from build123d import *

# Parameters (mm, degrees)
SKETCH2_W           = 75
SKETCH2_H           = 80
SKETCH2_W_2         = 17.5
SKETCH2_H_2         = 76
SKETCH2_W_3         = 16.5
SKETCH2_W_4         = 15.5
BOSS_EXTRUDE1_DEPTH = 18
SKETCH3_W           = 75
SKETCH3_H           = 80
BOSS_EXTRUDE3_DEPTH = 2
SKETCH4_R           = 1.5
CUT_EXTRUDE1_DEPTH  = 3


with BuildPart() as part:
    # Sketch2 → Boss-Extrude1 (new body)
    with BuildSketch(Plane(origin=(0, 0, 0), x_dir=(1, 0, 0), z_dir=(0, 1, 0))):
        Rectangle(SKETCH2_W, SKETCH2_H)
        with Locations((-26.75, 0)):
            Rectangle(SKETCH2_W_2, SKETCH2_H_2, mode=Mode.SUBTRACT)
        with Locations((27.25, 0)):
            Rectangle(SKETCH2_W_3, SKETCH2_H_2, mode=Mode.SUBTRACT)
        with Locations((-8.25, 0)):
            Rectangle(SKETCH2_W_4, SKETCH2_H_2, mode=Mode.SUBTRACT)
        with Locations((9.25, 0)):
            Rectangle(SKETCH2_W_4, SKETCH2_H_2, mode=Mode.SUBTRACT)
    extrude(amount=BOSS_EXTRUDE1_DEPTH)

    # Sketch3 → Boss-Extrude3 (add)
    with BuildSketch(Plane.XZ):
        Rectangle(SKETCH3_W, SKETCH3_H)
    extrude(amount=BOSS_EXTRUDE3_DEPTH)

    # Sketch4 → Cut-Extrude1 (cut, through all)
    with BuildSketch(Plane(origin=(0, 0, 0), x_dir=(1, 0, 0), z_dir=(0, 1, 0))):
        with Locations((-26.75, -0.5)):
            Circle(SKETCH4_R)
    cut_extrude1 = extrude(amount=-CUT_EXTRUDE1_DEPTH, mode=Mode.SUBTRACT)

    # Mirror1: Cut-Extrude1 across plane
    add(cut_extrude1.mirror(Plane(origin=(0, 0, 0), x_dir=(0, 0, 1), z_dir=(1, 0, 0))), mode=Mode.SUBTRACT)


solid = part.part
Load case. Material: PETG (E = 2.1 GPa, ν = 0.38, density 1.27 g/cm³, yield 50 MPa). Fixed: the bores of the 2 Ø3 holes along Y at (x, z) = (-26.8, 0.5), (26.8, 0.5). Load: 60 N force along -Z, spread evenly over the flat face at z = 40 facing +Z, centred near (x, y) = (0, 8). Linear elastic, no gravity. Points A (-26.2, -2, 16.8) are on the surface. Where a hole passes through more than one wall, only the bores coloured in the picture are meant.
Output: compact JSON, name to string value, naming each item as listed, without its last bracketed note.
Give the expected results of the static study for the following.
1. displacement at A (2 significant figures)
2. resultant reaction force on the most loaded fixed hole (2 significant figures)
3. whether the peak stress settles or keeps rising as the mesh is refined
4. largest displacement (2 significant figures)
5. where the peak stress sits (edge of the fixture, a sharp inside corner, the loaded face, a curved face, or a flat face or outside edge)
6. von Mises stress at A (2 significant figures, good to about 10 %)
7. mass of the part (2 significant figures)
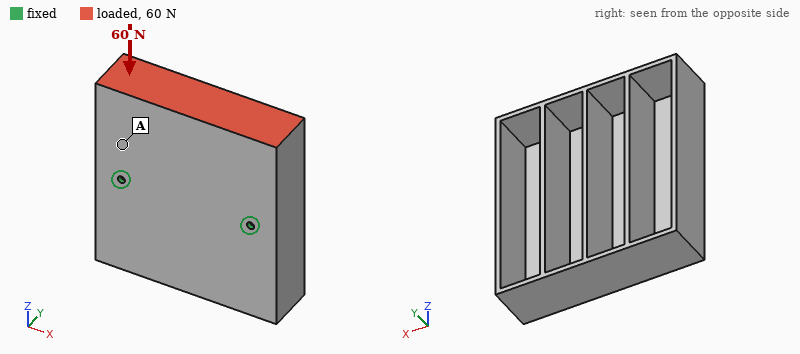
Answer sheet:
{"displacement at A": "0.35 mm", "resultant reaction force on the most loaded fixed hole": "30 N", "whether the peak stress settles or keeps rising as the mesh is refined": "keeps rising", "largest displacement": "1.0 mm", "where the peak stress sits": "edge of the fixture", "von Mises stress at A": "1.2 MPa", "mass of the part": "39 g"}
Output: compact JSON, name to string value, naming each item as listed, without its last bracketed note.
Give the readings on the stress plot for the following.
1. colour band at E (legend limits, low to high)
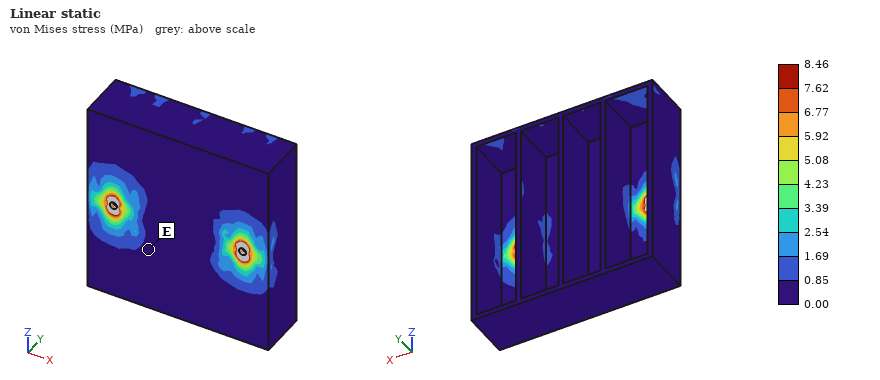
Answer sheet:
{"colour band at E": "0.00 to 0.85 MPa"}
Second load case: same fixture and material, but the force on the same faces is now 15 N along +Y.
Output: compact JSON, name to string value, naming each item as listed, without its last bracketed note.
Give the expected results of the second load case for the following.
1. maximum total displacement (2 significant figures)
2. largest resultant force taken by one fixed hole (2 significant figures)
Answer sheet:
{"maximum total displacement": "1.1 mm", "largest resultant force taken by one fixed hole": "7.6 N"}
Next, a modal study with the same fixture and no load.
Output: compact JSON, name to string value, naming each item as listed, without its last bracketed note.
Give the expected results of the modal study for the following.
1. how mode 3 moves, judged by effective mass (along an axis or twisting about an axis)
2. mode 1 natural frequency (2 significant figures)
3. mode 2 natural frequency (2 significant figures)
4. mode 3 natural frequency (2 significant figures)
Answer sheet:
{"how mode 3 moves, judged by effective mass": "along Y", "mode 1 natural frequency": "140 Hz", "mode 2 natural frequency": "310 Hz", "mode 3 natural frequency": "660 Hz"}
